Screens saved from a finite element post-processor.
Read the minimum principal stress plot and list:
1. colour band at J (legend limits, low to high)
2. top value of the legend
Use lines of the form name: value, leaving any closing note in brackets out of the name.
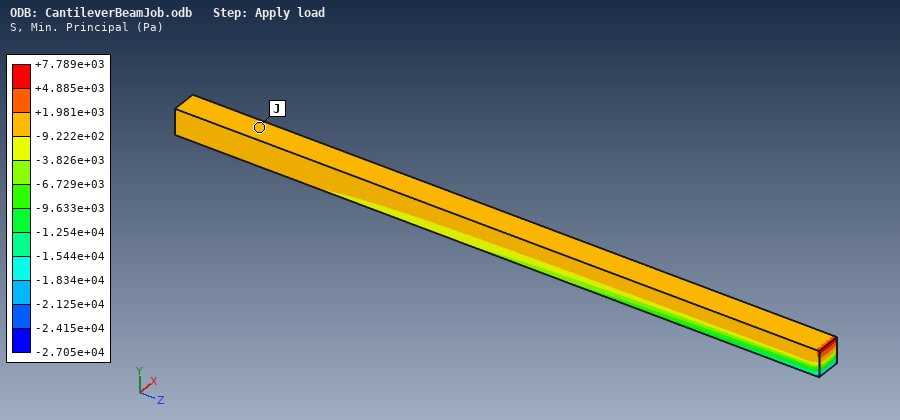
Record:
colour band at J: -9.222e+02 to +1.981e+03 Pa
top value of the legend: +7.789e+03 Pa
